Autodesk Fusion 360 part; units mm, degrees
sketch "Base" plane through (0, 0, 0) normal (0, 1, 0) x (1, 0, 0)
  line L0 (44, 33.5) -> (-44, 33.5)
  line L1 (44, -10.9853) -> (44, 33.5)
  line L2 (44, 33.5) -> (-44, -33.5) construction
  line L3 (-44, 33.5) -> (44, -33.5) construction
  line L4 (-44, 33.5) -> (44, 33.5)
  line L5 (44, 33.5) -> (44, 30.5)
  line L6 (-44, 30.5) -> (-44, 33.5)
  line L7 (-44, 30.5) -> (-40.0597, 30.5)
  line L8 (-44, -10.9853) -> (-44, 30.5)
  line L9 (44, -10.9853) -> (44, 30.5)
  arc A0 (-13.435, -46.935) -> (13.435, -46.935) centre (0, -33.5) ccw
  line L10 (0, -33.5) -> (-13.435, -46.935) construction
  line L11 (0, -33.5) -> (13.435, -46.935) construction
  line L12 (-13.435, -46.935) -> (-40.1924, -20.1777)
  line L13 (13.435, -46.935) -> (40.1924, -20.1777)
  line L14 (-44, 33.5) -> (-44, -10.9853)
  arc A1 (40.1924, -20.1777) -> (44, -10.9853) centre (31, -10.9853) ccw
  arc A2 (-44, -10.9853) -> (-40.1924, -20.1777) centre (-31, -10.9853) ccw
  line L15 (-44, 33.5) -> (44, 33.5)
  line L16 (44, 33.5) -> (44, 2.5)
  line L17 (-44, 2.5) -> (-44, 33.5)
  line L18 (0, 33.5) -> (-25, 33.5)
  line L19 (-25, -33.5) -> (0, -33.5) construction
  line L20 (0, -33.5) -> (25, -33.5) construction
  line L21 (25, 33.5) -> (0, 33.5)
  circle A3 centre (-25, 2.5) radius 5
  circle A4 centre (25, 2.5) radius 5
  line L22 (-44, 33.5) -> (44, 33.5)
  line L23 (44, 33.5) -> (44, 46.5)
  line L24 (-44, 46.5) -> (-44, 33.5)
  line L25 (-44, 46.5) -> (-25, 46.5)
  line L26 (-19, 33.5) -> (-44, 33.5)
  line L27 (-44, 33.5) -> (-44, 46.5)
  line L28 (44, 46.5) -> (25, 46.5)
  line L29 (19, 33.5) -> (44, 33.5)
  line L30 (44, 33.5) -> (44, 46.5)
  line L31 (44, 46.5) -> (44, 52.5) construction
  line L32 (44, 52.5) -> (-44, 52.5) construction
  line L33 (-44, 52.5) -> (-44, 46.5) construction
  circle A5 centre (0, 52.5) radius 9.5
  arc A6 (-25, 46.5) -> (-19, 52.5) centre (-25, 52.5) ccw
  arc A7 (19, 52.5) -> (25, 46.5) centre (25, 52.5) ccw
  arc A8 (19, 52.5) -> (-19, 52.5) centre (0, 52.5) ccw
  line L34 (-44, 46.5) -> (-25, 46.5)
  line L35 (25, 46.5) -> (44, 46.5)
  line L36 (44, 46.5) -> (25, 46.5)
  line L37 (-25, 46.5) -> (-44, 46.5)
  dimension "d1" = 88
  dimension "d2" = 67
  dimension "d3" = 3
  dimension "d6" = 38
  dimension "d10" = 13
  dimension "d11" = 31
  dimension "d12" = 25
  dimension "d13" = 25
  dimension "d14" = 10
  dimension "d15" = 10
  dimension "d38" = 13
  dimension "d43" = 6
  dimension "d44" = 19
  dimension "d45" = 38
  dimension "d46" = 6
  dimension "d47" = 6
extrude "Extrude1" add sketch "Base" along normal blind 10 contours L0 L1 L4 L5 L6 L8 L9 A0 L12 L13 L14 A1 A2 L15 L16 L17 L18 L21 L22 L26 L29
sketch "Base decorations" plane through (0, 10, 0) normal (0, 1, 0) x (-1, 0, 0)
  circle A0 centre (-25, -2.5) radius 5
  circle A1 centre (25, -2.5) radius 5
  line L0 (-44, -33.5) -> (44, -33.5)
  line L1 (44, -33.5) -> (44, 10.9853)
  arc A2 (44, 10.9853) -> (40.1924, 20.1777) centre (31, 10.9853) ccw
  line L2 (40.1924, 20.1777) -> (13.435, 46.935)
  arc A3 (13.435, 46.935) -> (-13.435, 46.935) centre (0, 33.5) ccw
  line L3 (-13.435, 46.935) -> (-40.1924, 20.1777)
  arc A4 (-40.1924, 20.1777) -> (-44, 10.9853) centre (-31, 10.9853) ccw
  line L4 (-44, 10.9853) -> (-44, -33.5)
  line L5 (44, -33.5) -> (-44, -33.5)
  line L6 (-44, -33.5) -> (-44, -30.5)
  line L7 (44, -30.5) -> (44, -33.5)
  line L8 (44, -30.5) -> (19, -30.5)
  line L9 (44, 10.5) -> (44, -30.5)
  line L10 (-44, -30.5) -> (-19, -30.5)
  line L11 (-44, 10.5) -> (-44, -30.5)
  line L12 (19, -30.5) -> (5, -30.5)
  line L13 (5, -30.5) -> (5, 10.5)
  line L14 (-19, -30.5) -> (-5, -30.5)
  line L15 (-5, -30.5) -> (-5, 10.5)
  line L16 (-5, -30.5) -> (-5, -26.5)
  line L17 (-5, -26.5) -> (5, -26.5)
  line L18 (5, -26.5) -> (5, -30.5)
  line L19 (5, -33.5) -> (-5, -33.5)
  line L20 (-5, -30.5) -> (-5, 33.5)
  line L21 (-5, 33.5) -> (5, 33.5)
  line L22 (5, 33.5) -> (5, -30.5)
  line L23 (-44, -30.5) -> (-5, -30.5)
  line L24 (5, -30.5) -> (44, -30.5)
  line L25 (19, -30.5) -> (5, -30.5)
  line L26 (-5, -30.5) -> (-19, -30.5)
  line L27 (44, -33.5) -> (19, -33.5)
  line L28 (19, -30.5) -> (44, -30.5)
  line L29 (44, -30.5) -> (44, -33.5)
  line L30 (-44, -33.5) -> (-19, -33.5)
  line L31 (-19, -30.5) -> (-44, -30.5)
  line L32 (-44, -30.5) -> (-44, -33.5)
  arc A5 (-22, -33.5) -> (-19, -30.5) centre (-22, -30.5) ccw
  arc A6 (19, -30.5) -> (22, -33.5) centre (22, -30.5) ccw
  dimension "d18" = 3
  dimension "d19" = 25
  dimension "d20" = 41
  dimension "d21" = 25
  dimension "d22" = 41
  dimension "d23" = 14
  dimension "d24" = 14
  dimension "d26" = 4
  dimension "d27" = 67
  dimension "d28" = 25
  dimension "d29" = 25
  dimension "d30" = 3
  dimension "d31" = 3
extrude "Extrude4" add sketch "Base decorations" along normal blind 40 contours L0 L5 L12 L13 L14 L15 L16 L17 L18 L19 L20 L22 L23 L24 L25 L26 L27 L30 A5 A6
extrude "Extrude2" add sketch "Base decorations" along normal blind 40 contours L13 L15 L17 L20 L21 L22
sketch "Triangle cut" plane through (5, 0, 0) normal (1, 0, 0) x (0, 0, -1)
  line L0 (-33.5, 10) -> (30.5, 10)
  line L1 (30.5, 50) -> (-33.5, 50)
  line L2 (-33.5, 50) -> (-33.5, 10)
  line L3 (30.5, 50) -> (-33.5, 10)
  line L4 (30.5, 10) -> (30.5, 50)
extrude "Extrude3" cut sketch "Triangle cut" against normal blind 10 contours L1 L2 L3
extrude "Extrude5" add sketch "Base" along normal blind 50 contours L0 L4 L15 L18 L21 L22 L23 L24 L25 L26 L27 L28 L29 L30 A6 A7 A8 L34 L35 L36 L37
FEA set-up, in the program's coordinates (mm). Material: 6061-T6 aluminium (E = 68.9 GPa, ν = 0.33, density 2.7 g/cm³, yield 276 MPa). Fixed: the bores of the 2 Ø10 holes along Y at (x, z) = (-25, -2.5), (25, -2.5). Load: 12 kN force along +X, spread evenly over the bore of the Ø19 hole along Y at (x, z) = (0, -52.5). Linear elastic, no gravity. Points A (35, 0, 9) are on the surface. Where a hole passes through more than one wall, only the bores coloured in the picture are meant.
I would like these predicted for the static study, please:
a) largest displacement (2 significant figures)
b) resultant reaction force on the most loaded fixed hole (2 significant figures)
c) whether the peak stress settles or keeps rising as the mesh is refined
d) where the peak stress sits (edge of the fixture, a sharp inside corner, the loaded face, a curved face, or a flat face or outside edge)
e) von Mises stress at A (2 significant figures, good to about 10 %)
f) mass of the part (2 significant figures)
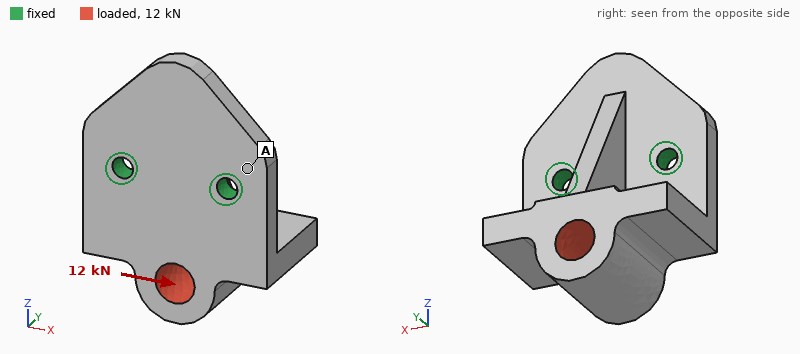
0.17 mm
13 kN
keeps rising
edge of the fixture
26 MPa
440 g
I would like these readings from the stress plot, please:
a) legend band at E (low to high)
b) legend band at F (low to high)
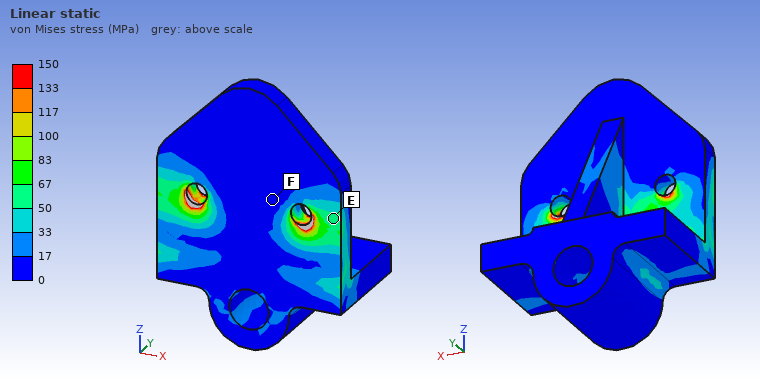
50 to 67 MPa
0 to 17 MPa
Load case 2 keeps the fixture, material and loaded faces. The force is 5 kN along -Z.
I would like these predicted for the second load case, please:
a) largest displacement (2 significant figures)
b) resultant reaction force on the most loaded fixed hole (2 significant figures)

0.14 mm
2.5 kN
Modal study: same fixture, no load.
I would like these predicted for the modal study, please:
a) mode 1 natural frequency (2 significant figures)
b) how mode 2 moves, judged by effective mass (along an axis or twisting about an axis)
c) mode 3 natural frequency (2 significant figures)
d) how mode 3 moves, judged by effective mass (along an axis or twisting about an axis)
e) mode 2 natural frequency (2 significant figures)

1600 Hz
along X
5200 Hz
along Y
2800 Hz
